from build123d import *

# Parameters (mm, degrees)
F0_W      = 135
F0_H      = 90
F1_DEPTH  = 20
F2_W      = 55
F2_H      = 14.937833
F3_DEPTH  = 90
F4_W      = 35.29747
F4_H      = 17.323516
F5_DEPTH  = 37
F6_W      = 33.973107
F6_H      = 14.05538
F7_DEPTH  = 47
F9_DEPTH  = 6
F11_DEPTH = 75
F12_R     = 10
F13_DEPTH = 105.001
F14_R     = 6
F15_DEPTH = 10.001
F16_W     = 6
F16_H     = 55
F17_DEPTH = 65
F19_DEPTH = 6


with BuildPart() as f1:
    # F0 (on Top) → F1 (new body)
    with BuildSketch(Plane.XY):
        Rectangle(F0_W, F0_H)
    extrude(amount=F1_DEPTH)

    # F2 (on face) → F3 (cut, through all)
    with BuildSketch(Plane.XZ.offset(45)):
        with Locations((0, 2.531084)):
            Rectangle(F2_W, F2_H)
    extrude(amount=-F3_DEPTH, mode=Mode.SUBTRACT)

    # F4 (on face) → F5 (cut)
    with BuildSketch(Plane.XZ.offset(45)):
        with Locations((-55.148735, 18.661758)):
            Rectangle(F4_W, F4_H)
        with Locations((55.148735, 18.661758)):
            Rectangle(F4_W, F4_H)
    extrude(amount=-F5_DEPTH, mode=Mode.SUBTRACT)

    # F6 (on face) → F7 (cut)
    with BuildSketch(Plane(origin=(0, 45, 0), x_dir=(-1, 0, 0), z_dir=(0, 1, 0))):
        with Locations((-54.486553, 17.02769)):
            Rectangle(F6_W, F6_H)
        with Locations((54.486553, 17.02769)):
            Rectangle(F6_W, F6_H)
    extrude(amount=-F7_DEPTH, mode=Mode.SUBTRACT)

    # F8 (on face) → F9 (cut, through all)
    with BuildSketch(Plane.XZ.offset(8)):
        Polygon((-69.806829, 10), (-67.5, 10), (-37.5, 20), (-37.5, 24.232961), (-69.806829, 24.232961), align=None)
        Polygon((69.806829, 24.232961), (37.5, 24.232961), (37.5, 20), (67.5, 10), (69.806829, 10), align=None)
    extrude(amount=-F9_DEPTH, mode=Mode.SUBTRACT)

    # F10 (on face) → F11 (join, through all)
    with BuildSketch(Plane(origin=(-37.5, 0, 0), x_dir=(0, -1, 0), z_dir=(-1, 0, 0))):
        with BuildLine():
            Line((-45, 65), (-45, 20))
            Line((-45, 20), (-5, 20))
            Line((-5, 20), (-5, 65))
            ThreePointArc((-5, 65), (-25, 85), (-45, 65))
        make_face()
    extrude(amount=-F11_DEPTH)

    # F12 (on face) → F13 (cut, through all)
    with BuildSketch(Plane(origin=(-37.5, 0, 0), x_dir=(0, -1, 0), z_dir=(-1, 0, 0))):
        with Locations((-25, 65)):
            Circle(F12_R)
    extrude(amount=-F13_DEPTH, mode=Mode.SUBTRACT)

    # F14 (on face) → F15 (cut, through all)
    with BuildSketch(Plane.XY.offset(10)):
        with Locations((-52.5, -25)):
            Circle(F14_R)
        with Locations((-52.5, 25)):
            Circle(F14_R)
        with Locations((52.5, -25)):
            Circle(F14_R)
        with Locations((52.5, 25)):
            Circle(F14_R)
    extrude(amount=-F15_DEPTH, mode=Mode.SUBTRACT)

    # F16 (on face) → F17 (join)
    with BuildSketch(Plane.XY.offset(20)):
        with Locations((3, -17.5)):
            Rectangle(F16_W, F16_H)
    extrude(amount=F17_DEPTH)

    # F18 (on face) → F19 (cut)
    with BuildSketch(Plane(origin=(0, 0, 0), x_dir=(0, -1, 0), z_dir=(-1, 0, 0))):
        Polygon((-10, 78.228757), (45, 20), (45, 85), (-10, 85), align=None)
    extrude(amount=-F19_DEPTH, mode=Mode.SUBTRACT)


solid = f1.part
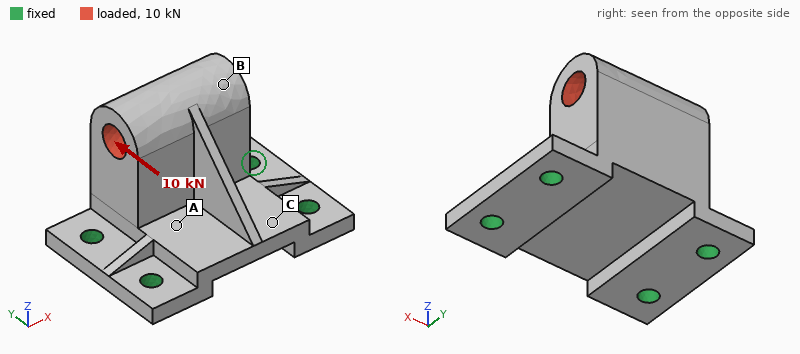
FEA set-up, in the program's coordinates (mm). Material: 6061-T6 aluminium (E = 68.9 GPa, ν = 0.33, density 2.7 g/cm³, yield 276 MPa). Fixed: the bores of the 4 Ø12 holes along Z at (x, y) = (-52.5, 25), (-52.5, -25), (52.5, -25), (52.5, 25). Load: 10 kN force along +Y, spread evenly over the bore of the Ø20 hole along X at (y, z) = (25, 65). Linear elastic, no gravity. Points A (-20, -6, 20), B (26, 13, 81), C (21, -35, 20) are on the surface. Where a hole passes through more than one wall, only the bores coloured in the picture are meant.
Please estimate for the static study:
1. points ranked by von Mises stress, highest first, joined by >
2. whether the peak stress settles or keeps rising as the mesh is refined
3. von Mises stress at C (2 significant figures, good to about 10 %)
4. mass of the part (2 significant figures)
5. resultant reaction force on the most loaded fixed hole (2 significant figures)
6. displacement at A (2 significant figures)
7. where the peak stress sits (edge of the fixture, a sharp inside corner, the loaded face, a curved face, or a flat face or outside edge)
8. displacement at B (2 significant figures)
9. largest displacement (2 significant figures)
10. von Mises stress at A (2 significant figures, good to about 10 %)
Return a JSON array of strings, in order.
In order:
["A > C > B", "keeps rising", "23 MPa", "820 g", "9.7 kN", "0.034 mm", "edge of the fixture", "0.17 mm", "0.18 mm", "32 MPa"]
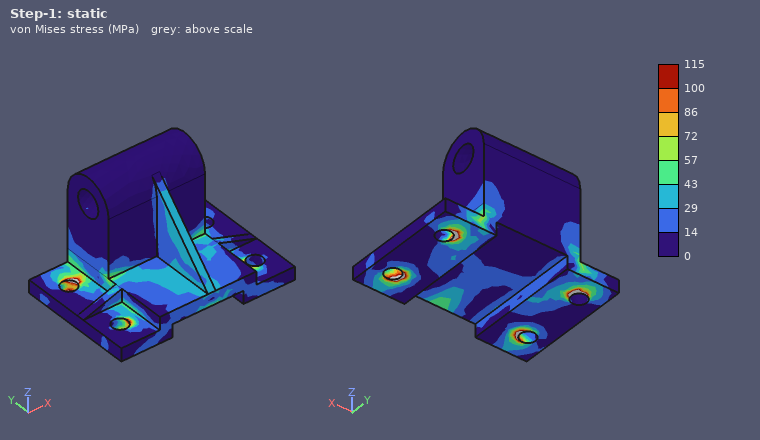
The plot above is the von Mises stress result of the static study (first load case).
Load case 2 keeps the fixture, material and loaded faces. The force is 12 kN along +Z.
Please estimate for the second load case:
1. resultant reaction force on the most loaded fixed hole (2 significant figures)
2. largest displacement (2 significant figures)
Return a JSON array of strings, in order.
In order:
["6.9 kN", "52 µm"]
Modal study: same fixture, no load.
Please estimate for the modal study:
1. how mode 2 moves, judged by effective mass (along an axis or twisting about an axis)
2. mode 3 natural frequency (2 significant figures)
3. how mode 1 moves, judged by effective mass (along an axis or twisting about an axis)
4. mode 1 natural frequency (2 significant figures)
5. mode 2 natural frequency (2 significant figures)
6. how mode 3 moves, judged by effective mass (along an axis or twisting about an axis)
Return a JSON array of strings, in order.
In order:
["along X", "4800 Hz", "along Y", "2400 Hz", "4100 Hz", "along Z"]
